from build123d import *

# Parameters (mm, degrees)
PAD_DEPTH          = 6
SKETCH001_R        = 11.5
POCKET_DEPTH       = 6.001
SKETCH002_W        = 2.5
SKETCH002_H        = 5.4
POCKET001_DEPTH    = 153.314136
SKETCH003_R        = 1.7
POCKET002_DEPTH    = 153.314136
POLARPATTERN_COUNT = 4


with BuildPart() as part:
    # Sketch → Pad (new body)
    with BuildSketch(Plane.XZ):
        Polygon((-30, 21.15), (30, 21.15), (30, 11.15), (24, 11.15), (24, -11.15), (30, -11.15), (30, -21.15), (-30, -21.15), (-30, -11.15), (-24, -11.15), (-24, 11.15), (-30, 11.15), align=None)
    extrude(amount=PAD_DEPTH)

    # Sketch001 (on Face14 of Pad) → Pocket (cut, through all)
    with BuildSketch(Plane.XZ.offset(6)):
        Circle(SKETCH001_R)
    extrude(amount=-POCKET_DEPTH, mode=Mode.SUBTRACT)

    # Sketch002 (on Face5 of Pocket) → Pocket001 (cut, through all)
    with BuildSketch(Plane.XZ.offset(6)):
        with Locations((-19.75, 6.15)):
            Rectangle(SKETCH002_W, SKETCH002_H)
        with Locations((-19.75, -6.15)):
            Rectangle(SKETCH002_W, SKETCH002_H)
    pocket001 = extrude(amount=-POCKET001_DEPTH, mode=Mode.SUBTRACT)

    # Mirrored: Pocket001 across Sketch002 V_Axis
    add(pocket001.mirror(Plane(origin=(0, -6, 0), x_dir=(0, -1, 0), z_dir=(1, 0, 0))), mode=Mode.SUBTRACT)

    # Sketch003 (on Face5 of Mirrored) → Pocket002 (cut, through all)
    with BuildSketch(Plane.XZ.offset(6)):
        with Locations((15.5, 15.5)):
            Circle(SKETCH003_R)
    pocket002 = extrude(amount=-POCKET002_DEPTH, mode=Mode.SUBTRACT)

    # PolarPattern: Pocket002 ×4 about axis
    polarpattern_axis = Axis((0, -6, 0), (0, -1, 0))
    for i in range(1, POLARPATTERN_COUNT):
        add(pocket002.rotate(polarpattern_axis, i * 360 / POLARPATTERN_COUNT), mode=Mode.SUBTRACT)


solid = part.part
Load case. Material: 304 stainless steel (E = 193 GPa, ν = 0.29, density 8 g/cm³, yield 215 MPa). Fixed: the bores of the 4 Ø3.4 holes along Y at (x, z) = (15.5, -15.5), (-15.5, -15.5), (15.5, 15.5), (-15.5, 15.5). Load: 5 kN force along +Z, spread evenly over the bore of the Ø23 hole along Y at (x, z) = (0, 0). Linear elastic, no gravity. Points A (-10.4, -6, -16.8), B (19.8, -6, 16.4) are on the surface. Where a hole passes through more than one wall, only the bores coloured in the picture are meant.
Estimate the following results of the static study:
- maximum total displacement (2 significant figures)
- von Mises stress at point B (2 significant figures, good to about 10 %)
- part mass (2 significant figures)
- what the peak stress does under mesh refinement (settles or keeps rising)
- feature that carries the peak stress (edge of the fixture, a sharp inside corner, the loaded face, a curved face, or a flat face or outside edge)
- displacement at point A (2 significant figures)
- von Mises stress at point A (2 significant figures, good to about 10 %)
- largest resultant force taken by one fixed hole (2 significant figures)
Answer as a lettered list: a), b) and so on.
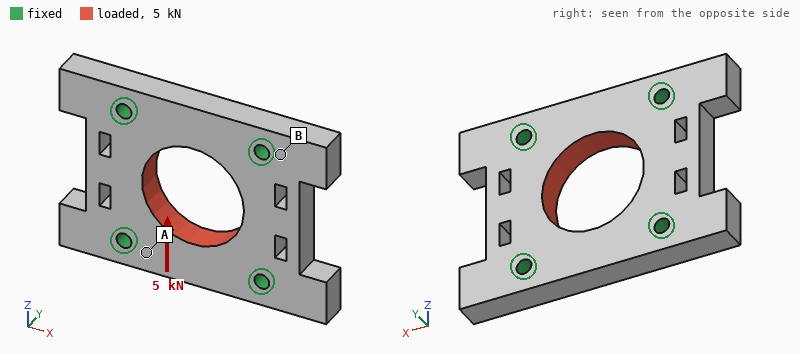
a) 2.7 µm
b) 6.7 MPa
c) 85 g
d) keeps rising
e) edge of the fixture
f) 0.98 µm
g) 16 MPa
h) 1.3 kN
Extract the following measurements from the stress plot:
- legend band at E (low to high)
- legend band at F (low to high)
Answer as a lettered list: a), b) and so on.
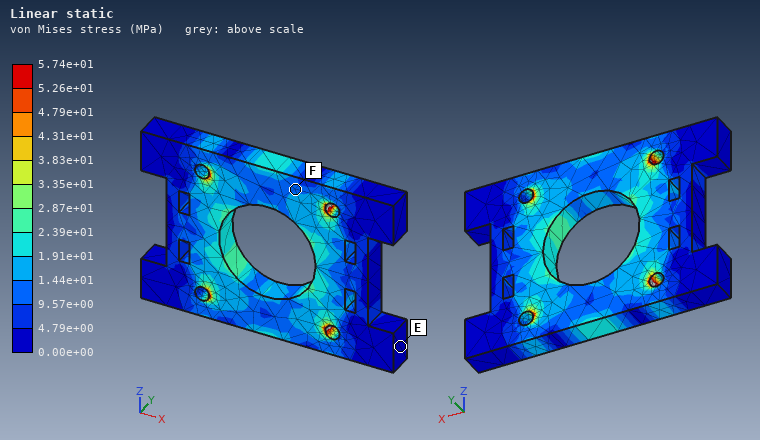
a) 0.00e+00 to 4.79e+00 MPa
b) 9.57e+00 to 1.44e+01 MPa
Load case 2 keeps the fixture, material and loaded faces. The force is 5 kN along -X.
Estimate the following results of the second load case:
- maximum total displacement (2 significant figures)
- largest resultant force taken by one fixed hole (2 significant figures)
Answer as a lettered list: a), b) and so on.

a) 2.7 µm
b) 1.3 kN
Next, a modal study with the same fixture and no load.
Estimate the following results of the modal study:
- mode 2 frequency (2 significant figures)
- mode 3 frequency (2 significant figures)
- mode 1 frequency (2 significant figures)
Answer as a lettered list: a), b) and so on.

a) 21 kHz
b) 23 kHz
c) 21 kHz
